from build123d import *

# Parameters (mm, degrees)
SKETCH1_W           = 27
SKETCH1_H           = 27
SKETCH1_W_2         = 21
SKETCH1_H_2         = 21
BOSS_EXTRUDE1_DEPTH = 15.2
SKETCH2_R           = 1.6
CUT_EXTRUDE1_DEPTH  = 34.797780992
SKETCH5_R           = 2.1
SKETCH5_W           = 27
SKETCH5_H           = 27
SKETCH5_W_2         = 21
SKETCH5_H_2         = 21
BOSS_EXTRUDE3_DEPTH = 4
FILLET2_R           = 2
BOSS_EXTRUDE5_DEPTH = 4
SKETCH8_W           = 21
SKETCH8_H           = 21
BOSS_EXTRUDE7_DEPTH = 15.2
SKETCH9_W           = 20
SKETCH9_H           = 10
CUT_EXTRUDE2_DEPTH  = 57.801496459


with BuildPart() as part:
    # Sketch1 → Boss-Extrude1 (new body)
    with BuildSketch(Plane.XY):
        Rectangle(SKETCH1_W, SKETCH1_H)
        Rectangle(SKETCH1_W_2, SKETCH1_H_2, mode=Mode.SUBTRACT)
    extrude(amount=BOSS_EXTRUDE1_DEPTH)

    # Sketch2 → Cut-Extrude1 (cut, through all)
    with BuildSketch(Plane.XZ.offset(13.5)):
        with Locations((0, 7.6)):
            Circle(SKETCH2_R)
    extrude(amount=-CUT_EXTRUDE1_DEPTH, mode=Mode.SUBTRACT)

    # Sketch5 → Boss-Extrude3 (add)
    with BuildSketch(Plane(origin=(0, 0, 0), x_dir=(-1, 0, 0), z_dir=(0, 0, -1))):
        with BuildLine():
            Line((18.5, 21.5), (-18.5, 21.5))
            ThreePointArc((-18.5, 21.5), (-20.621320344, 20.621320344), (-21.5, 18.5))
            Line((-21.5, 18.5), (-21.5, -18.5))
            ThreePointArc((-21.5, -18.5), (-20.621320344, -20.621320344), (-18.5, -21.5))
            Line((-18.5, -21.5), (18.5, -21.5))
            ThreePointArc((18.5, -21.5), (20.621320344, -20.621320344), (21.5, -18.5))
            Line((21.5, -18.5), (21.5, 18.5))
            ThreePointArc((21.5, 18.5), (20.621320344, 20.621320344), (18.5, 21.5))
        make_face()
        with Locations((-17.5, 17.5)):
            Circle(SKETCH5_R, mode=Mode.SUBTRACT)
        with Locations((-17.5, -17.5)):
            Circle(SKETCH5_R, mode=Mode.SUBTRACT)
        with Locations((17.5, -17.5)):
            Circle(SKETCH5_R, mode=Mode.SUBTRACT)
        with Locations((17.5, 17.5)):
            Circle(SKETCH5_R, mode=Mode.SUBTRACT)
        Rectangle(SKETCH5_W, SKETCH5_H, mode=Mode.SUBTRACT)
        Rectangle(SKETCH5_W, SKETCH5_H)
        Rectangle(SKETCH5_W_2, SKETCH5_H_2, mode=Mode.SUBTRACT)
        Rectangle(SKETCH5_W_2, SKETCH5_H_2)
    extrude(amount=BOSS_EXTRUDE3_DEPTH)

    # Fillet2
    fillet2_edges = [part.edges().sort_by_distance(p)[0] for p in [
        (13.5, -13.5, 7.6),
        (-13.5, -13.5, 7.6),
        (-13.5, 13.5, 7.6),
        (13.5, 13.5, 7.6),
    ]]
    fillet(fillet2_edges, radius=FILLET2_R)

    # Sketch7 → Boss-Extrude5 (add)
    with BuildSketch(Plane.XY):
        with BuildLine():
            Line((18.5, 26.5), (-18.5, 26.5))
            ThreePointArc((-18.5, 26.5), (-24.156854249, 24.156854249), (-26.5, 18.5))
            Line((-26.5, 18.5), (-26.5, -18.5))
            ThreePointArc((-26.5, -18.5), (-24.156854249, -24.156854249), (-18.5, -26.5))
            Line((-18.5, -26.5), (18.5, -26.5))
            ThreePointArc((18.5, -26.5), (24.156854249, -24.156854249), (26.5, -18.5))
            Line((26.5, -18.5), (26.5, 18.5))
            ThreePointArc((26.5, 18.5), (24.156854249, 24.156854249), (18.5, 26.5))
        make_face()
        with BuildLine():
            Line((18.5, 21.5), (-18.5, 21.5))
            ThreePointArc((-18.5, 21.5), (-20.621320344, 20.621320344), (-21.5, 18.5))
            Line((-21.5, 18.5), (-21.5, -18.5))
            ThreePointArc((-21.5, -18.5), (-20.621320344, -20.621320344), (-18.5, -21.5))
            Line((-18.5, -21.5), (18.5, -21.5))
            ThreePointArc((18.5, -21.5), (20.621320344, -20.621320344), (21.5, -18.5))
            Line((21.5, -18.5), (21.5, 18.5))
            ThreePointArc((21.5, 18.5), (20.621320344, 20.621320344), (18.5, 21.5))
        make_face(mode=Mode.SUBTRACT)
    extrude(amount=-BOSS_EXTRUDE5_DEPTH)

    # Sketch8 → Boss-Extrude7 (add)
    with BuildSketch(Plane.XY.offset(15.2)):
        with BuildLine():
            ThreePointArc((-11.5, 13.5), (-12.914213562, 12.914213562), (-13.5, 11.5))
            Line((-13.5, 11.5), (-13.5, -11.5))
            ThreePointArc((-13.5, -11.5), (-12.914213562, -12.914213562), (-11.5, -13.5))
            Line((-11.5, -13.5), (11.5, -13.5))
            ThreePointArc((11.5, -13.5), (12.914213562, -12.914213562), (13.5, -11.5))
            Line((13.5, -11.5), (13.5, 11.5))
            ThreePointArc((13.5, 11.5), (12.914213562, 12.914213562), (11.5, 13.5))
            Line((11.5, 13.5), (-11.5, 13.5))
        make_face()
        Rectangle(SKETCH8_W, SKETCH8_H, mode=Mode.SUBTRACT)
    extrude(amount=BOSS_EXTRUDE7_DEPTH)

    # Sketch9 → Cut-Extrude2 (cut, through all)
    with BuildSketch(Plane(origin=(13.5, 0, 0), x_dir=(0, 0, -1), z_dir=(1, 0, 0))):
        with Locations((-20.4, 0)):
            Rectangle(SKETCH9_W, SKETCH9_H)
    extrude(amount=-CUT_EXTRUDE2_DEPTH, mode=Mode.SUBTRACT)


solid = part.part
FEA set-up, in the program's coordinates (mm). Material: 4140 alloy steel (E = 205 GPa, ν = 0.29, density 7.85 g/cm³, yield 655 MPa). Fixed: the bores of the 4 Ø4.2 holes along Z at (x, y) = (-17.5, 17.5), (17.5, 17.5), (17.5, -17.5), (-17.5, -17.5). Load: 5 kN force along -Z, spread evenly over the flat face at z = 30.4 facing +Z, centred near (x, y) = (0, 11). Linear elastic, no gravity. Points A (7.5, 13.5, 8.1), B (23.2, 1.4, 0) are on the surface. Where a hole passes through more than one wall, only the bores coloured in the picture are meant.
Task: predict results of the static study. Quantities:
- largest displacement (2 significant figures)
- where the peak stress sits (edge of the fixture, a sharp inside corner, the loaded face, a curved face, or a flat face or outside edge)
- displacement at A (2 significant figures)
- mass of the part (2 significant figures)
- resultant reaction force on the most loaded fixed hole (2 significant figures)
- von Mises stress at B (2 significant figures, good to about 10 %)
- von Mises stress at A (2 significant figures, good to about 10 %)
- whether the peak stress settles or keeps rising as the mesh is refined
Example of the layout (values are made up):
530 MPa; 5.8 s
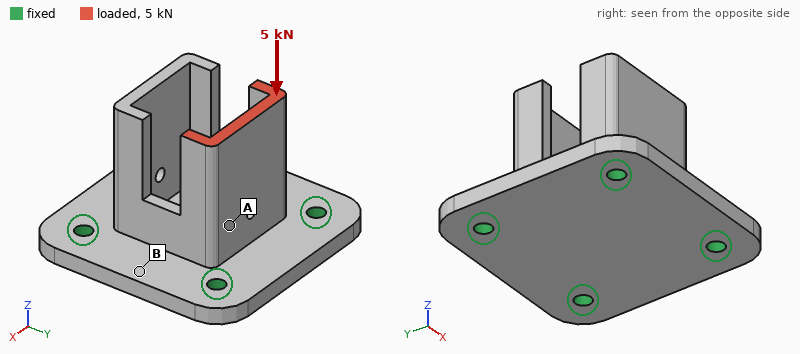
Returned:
27 µm; edge of the fixture; 16 µm; 140 g; 2.2 kN; 23 MPa; 56 MPa; keeps rising
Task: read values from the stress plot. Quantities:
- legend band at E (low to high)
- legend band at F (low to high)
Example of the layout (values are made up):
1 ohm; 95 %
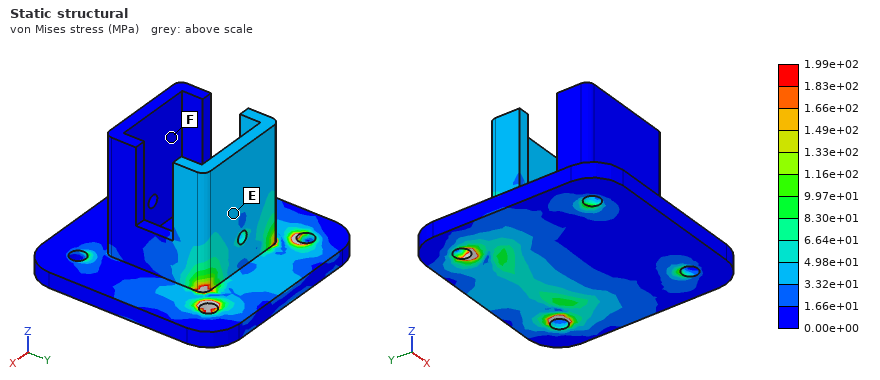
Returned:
3.32e+01 to 4.98e+01 MPa; 0.00e+00 to 1.66e+01 MPa
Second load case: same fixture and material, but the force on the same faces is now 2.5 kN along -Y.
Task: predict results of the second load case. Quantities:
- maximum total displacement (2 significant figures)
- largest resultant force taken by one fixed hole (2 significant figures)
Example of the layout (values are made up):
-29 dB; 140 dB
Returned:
0.21 mm; 1.7 kN
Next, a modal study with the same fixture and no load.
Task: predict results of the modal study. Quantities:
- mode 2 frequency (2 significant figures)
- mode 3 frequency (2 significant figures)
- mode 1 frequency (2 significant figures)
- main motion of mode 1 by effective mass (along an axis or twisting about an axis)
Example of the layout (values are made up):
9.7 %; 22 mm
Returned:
7600 Hz; 8800 Hz; 6900 Hz; along Y
